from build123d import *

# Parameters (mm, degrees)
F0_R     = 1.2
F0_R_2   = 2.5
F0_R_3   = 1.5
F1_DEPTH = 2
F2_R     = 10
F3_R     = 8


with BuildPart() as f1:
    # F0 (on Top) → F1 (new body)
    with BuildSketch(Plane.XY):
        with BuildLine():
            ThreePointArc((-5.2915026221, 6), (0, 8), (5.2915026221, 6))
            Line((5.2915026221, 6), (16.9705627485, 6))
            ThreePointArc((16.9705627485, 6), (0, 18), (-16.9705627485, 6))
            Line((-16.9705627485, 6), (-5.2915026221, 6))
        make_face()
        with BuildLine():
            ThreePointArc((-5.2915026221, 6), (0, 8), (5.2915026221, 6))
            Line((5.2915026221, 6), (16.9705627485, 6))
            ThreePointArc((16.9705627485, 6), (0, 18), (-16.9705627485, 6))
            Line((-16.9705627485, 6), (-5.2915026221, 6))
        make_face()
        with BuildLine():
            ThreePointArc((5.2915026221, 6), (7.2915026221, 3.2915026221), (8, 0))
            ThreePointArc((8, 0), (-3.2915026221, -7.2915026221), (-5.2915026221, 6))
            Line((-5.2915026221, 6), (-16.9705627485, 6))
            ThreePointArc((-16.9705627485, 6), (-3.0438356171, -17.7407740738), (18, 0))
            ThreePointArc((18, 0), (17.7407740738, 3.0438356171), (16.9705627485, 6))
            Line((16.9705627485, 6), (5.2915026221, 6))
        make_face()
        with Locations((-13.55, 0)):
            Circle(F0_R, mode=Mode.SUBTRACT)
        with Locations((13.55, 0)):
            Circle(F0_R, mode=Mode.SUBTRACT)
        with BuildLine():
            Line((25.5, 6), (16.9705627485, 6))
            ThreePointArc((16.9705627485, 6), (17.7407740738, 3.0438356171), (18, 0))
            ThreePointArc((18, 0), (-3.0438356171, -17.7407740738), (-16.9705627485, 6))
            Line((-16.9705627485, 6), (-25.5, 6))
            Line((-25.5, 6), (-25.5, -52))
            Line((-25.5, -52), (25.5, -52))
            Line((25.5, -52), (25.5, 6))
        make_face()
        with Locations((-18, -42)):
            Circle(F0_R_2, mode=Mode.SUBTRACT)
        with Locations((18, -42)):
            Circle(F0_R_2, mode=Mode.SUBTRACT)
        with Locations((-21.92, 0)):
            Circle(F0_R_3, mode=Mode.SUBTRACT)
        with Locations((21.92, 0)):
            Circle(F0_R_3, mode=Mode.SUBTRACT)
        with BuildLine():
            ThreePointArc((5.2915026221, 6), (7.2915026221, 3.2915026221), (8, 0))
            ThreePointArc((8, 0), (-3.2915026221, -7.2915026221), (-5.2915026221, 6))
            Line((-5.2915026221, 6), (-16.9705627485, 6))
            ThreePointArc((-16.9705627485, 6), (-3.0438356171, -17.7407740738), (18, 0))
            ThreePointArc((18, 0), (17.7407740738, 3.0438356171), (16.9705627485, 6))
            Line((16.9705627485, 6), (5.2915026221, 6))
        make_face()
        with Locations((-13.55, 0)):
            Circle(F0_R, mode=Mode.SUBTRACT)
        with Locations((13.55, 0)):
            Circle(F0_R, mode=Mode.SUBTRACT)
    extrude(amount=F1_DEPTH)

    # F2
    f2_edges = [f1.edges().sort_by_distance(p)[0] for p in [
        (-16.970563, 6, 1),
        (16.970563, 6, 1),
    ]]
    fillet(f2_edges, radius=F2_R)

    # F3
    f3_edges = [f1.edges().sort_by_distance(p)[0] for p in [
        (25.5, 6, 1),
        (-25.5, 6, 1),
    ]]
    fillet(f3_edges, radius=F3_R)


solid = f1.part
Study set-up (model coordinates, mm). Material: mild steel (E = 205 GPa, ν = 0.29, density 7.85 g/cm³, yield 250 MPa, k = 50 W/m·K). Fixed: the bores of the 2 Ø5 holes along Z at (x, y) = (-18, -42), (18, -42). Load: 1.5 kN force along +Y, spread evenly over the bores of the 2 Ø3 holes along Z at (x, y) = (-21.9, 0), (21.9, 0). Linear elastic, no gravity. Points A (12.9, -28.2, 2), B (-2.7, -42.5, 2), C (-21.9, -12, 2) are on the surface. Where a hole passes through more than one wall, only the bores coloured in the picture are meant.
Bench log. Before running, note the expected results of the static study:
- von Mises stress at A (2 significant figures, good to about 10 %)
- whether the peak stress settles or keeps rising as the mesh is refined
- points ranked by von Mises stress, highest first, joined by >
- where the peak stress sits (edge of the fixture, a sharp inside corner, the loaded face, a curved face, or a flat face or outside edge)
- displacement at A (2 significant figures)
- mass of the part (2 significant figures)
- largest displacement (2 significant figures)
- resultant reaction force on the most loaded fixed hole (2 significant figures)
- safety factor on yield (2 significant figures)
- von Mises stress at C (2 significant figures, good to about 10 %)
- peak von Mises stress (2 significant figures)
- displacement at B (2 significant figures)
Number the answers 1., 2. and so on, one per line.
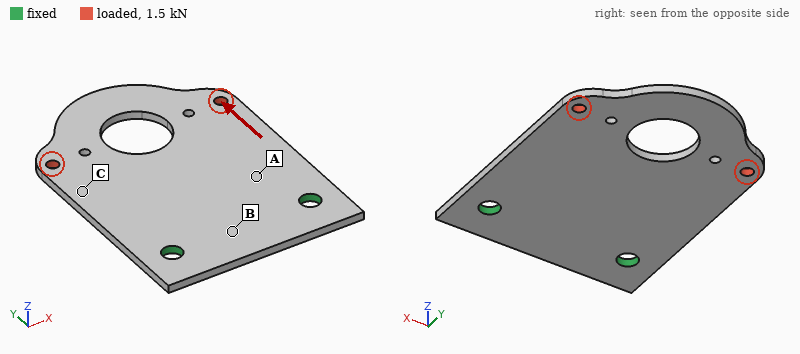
1. 15 MPa
2. settles
3. C > A > B
4. the loaded face
5. 1.5 µm
6. 47 g
7. 6.0 µm
8. 750 N
9. 2.5
10. 26 MPa
11. 100 MPa
12. 1.3 µm
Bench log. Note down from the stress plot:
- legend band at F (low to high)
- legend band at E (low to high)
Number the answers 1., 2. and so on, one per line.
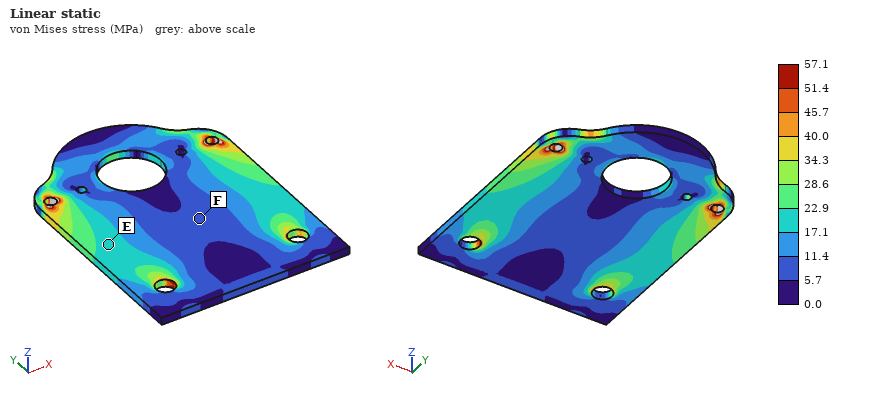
1. 5.7 to 11.4 MPa
2. 17.1 to 22.9 MPa
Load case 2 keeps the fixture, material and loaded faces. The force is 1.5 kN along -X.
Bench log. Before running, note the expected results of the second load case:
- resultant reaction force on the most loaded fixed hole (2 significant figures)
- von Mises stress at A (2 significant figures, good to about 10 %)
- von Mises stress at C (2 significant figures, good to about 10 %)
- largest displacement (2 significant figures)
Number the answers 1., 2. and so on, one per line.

1. 1.8 kN
2. 37 MPa
3. 27 MPa
4. 27 µm
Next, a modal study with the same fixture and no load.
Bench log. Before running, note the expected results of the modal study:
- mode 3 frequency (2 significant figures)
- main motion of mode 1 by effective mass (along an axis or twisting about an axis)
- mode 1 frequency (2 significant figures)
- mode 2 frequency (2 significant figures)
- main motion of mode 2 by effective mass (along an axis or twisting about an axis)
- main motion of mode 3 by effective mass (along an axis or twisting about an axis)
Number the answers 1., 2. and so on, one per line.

1. 3000 Hz
2. along Z
3. 610 Hz
4. 1700 Hz
5. twisting about Y
6. along Z
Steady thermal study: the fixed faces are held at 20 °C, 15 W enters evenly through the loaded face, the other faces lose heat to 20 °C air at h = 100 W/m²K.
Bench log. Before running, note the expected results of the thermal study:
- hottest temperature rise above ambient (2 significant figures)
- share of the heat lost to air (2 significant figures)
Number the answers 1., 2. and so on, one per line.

1. 79 K
2. 82 %
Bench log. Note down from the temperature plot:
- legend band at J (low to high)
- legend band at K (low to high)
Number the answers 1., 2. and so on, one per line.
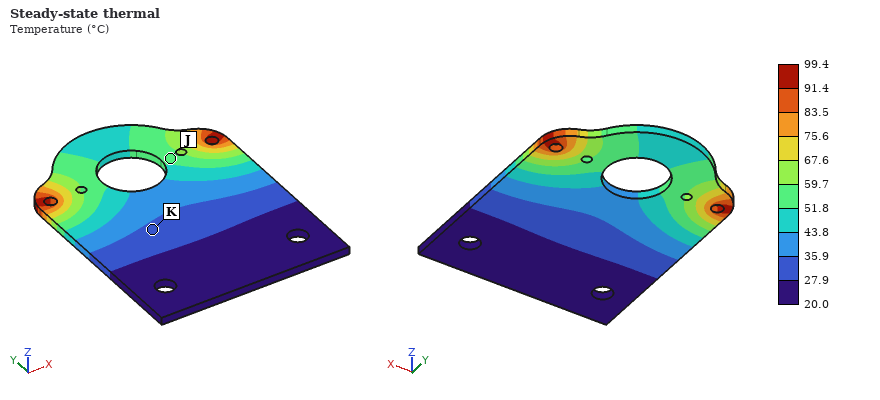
1. 51.8 to 59.7 °C
2. 27.9 to 35.9 °C
